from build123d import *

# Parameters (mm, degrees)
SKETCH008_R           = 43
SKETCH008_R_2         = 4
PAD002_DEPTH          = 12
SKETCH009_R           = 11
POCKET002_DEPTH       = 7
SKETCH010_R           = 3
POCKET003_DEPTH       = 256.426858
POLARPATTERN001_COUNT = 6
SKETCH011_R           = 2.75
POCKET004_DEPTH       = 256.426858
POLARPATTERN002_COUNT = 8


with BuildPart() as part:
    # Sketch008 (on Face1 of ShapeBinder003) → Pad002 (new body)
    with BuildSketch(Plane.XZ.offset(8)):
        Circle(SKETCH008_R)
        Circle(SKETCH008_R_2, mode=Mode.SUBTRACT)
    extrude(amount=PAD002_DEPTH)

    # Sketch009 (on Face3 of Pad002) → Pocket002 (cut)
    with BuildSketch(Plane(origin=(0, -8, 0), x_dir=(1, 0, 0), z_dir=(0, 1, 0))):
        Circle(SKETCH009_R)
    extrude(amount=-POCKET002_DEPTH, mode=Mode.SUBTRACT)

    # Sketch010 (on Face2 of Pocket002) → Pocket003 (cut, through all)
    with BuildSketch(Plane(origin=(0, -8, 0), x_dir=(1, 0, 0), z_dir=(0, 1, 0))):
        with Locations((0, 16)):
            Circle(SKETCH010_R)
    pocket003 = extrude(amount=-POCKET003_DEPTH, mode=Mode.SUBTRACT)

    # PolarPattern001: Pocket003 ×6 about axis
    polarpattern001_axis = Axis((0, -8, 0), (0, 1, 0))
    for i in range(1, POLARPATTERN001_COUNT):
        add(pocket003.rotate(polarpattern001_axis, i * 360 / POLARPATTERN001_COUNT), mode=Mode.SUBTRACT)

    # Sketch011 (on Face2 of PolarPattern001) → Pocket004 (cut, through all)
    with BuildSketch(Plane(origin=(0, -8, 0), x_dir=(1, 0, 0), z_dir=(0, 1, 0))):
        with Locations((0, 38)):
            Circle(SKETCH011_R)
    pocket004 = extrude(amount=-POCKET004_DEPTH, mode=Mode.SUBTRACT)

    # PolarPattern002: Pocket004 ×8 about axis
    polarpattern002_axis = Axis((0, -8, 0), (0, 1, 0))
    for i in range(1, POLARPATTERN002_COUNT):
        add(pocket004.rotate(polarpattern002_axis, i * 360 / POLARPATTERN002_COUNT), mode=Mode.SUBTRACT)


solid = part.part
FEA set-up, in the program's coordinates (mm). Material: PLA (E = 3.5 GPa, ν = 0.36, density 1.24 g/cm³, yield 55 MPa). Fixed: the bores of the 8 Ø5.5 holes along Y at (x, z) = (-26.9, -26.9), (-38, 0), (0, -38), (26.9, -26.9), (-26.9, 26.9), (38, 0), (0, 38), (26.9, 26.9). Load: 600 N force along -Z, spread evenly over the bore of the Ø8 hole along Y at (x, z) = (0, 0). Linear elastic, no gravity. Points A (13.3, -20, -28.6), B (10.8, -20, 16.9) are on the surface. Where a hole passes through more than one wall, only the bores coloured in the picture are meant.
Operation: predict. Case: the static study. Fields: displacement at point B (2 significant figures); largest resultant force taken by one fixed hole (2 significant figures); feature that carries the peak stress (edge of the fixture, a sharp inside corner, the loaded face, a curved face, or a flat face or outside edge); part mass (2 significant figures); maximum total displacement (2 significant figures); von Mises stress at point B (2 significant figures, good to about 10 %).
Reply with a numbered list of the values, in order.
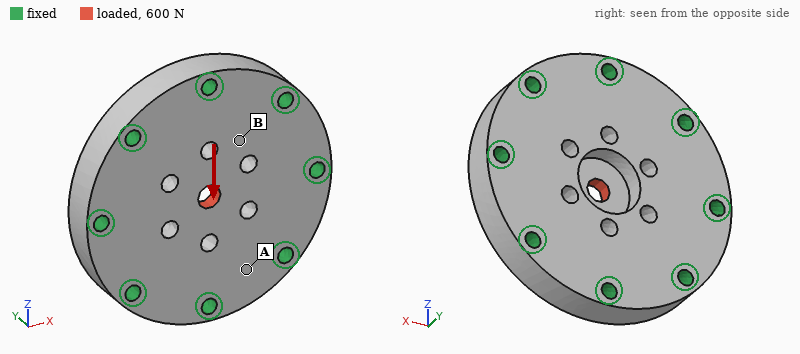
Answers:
1. 4.7 µm
2. 130 N
3. the loaded face
4. 77 g
5. 19 µm
6. 1.3 MPa
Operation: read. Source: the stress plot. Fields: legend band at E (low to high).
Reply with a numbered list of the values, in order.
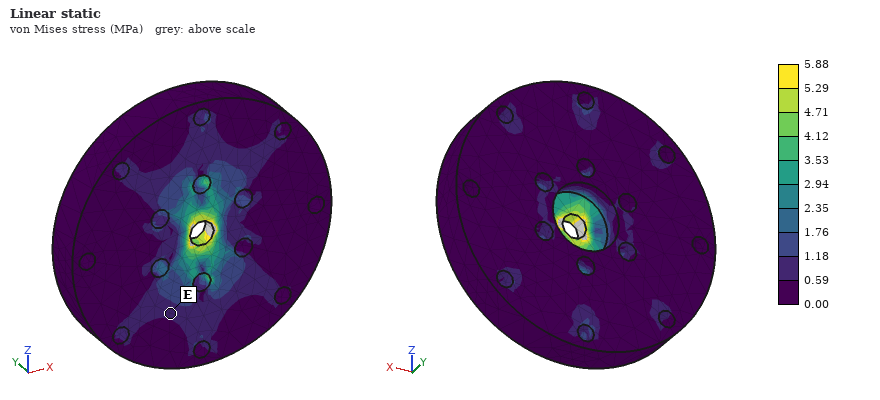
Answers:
1. 0.59 to 1.18 MPa
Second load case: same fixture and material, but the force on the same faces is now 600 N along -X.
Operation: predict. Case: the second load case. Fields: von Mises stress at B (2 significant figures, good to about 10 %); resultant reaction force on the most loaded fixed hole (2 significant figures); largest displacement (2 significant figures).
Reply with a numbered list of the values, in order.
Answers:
1. 0.86 MPa
2. 130 N
3. 19 µm
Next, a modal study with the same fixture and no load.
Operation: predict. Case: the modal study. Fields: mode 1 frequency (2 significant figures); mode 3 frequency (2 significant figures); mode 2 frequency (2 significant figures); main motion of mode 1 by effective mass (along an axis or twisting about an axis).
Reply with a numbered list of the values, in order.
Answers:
1. 5200 Hz
2. 8300 Hz
3. 8300 Hz
4. along Y
